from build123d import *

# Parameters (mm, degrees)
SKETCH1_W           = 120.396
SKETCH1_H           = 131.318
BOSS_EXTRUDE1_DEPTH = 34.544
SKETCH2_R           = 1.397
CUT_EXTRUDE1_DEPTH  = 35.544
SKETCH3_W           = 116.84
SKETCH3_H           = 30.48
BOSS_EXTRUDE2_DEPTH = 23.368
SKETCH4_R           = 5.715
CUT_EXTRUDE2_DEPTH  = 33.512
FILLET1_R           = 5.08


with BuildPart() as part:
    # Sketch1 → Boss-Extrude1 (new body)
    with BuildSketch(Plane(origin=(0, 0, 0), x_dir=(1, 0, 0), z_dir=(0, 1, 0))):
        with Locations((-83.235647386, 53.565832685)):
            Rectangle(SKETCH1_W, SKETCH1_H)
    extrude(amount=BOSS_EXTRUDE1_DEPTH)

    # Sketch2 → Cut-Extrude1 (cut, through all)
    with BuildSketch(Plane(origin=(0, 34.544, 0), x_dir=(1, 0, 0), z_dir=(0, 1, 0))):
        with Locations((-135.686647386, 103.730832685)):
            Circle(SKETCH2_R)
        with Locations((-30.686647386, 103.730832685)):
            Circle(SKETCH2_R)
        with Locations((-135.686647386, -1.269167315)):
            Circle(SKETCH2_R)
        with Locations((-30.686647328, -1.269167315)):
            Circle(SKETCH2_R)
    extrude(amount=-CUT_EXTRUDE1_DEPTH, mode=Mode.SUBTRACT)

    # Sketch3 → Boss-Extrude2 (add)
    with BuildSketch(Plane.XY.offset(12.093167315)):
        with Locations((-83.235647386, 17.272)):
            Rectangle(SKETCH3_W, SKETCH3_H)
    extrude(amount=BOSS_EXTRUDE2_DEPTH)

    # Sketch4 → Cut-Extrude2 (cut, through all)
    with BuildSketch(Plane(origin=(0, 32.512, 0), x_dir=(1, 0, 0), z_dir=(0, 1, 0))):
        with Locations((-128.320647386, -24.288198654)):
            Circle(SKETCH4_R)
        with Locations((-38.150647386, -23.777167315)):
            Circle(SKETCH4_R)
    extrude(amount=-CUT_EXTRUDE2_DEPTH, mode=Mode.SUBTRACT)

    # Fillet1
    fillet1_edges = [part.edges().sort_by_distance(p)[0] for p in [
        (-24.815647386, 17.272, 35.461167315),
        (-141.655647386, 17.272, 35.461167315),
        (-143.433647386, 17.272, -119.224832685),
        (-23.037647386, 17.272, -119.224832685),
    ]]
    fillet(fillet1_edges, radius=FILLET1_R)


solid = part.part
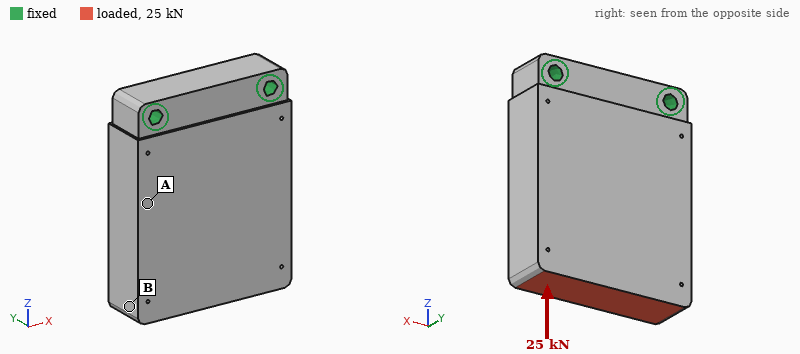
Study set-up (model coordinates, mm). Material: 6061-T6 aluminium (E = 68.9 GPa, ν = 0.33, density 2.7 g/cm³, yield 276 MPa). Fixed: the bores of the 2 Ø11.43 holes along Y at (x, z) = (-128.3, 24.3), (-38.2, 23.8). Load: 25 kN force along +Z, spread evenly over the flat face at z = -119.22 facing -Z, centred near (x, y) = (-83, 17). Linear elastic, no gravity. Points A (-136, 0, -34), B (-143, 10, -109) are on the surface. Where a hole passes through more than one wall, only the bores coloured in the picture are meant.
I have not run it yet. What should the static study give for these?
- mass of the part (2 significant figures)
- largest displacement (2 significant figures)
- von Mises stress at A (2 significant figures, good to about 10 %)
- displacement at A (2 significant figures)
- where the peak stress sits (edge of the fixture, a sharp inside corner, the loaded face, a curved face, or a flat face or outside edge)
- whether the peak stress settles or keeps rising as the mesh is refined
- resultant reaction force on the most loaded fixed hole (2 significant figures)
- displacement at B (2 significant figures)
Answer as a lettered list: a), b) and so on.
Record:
a) 1.7 kg
b) 16 µm
c) 6.8 MPa
d) 7.6 µm
e) edge of the fixture
f) keeps rising
g) 13 kN
h) 13 µm
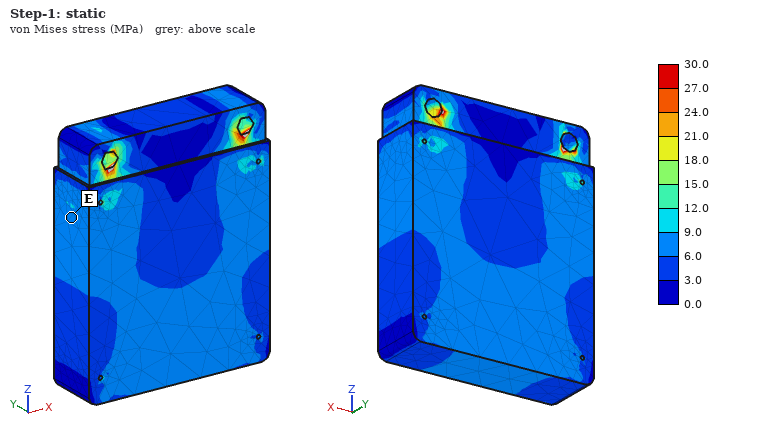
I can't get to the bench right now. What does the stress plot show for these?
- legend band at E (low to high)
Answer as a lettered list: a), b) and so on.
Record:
a) 6.0 to 9.0 MPa
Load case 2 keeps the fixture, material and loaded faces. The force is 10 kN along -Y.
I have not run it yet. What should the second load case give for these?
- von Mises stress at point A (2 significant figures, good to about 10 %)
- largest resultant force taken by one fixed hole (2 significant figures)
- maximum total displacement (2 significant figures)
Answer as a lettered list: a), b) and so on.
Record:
a) 37 MPa
b) 5.1 kN
c) 0.54 mm
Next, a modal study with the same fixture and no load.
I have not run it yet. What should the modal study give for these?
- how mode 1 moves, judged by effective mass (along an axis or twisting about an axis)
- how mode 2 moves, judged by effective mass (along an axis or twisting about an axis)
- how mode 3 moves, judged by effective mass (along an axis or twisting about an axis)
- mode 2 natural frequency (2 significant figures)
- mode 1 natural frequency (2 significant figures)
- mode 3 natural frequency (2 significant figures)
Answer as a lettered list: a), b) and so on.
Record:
a) along Y
b) twisting about Z
c) along X
d) 3100 Hz
e) 1000 Hz
f) 3200 Hz
